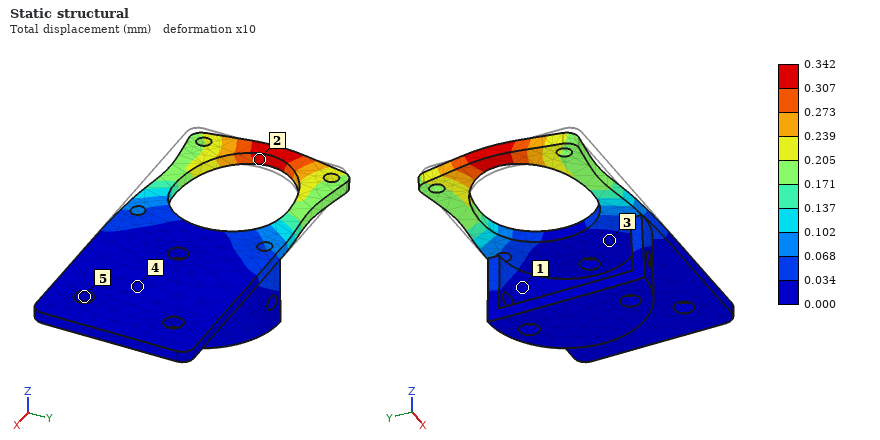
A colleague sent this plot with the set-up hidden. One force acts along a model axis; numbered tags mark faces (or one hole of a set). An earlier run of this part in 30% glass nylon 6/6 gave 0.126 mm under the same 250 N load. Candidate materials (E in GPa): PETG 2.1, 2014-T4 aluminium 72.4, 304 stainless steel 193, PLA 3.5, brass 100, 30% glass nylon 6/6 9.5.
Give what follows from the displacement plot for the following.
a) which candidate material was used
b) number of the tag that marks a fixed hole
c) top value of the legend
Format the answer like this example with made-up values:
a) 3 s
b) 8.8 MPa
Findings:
a) PLA
b) 5
c) 0.342 mm
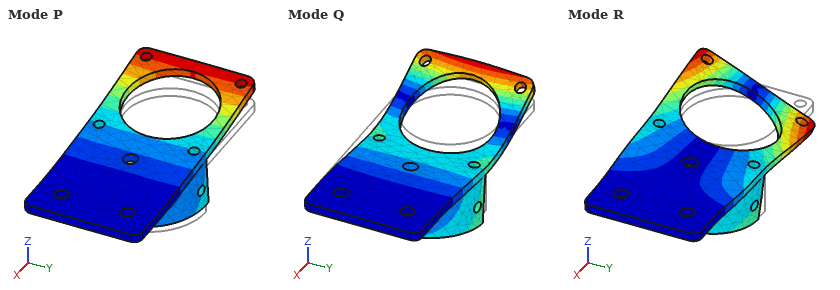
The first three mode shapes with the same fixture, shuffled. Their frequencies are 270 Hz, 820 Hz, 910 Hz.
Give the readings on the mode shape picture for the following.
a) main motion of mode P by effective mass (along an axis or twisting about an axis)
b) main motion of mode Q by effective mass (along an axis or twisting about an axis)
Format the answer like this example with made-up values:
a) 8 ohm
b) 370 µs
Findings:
a) along Z
b) along Z
